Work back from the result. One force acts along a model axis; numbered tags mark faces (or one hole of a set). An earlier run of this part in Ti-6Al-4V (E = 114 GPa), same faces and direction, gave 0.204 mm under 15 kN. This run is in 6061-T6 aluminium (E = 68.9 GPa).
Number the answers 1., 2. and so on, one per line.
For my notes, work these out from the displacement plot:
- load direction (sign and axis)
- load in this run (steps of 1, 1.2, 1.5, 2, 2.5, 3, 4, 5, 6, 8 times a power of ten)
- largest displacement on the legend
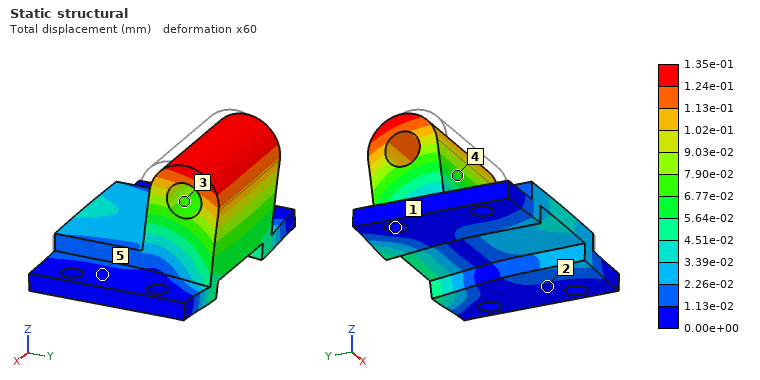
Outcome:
1. +Y
2. 6 kN
3. 1.35e-01 mm
